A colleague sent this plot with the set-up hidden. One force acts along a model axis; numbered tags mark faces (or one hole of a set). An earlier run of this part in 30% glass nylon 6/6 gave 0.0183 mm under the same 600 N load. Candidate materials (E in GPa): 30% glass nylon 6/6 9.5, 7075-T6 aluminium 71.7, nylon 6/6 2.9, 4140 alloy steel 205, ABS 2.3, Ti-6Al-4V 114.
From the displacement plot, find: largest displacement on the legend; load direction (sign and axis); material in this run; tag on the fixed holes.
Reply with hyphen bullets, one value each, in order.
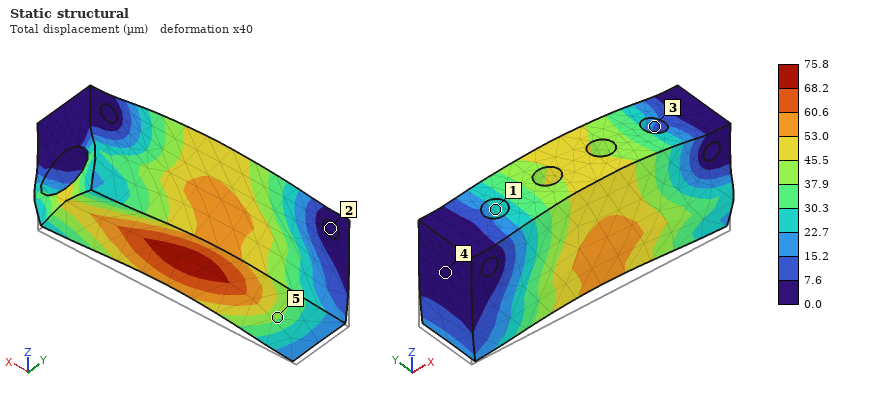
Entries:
- 75.8 µm
- +Z
- ABS
- 2
